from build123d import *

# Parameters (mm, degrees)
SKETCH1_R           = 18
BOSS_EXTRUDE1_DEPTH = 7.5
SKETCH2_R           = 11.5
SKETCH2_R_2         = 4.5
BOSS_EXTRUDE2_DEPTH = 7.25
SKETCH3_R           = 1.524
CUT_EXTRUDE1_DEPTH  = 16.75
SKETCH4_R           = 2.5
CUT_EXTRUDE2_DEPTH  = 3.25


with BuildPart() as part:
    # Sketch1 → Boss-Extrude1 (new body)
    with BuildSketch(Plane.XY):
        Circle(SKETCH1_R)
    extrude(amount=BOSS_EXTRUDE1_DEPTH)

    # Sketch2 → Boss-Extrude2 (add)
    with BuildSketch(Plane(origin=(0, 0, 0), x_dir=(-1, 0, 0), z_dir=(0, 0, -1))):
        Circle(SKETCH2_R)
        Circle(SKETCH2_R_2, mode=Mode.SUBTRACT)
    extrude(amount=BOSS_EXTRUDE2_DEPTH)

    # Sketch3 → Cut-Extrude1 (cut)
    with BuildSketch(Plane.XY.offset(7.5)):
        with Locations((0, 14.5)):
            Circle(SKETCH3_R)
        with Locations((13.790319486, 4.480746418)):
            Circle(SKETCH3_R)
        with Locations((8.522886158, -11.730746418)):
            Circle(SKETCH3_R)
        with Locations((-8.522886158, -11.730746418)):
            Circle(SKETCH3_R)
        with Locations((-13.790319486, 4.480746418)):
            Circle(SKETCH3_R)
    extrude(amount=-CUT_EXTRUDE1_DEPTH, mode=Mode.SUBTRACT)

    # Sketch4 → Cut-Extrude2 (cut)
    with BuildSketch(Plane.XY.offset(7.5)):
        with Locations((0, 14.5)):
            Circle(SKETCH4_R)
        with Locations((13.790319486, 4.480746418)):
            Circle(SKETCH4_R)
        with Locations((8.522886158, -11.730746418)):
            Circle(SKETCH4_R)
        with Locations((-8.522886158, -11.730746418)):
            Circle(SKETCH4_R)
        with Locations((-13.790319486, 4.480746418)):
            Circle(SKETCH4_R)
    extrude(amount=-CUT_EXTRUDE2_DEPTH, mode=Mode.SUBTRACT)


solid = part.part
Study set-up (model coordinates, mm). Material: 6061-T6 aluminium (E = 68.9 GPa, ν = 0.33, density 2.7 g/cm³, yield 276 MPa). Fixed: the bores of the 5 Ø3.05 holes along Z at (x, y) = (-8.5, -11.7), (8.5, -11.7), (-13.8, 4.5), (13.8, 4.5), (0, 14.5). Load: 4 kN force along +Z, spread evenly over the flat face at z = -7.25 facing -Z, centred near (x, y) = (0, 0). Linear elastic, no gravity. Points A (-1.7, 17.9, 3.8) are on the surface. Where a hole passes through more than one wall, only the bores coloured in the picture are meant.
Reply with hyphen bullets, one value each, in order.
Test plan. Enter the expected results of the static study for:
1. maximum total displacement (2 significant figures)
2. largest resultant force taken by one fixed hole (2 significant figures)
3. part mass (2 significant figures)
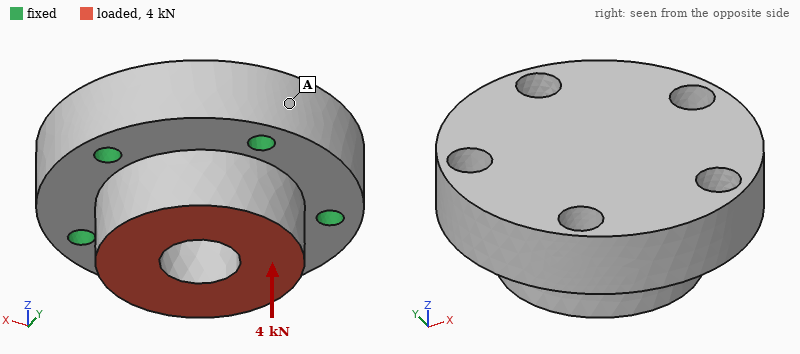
- 4.5 µm
- 800 N
- 26 g
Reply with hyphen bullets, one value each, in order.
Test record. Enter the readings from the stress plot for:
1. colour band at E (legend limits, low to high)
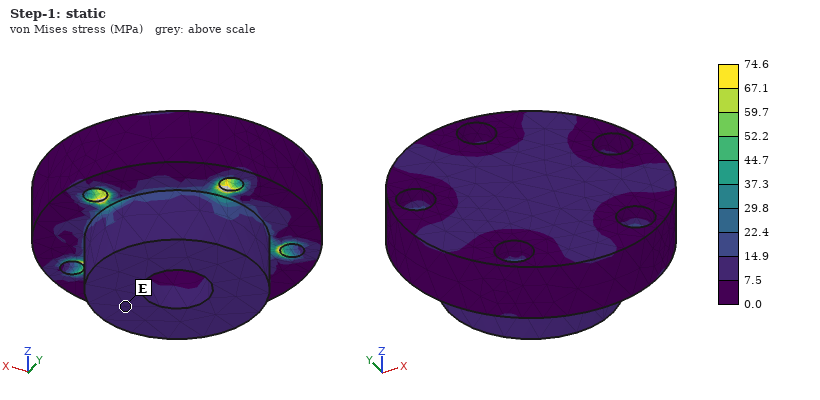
- 7.5 to 14.9 MPa
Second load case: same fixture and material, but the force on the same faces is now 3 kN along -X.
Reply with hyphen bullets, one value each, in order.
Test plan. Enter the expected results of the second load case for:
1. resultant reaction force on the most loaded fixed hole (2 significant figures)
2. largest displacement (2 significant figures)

- 1.0 kN
- 9.5 µm
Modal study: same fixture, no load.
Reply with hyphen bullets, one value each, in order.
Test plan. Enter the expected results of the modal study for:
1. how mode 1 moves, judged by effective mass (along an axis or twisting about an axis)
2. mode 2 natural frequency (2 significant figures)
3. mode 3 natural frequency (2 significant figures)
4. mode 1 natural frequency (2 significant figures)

- along Z
- 45 kHz
- 45 kHz
- 39 kHz
